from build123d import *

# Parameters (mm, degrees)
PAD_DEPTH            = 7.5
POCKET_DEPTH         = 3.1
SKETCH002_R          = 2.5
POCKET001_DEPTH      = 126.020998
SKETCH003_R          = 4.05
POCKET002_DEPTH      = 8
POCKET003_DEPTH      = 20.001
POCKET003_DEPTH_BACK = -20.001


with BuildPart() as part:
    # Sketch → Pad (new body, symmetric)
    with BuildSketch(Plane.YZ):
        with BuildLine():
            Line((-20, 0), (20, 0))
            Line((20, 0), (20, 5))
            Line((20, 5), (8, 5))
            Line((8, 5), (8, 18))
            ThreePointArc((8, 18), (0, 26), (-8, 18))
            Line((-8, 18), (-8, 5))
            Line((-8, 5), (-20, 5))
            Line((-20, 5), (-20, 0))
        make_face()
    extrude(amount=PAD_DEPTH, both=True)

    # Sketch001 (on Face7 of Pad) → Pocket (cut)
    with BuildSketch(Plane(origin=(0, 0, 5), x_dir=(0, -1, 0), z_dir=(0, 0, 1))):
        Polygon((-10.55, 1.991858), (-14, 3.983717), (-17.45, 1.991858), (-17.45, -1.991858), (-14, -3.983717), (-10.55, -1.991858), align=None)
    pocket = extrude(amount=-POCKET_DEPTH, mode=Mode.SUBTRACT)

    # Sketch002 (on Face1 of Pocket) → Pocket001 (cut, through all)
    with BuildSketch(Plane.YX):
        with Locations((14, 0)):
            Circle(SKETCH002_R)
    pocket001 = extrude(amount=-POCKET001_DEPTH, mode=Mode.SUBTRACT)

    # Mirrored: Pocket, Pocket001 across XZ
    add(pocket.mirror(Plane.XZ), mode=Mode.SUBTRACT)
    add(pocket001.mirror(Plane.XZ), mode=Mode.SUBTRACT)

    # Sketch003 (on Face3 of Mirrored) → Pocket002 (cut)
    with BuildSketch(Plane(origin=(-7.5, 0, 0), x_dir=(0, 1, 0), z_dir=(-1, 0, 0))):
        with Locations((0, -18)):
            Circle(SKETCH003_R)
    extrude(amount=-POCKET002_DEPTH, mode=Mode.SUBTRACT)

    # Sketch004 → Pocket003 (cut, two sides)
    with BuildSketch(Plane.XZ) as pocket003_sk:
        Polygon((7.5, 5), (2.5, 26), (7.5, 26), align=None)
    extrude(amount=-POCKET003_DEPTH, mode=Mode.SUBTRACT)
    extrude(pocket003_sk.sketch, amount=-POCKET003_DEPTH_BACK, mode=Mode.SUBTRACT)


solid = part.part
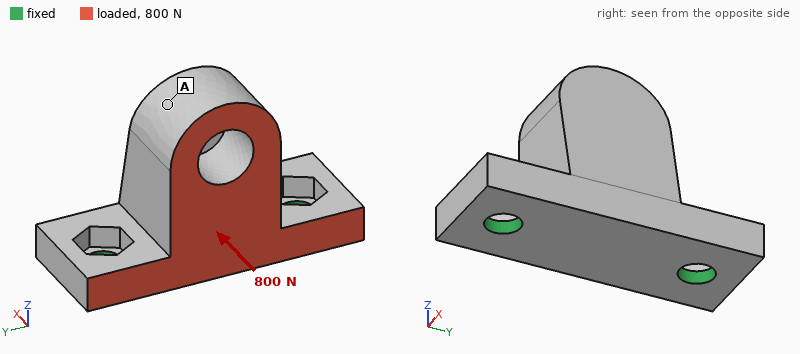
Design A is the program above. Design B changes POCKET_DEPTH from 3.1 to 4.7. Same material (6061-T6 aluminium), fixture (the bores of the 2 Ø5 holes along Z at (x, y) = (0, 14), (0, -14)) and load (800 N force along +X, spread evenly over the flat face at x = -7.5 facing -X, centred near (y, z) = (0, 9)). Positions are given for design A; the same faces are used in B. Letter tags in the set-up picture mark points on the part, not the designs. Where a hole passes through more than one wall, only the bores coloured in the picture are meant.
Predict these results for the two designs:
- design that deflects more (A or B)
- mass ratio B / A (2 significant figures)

B
0.99
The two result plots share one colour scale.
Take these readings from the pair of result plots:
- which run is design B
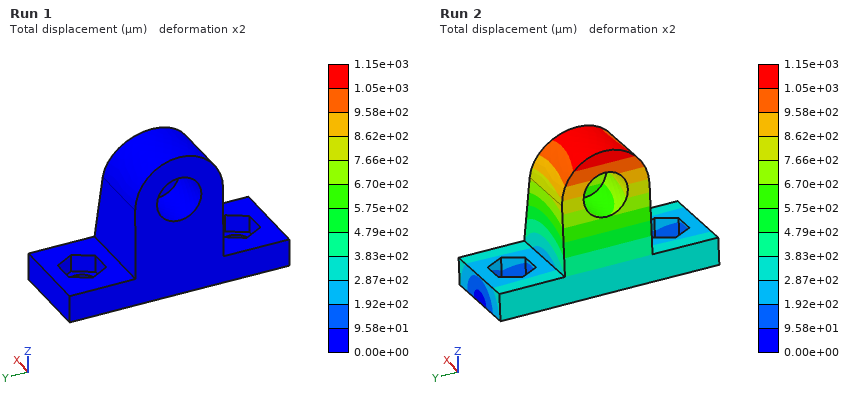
Run 2
